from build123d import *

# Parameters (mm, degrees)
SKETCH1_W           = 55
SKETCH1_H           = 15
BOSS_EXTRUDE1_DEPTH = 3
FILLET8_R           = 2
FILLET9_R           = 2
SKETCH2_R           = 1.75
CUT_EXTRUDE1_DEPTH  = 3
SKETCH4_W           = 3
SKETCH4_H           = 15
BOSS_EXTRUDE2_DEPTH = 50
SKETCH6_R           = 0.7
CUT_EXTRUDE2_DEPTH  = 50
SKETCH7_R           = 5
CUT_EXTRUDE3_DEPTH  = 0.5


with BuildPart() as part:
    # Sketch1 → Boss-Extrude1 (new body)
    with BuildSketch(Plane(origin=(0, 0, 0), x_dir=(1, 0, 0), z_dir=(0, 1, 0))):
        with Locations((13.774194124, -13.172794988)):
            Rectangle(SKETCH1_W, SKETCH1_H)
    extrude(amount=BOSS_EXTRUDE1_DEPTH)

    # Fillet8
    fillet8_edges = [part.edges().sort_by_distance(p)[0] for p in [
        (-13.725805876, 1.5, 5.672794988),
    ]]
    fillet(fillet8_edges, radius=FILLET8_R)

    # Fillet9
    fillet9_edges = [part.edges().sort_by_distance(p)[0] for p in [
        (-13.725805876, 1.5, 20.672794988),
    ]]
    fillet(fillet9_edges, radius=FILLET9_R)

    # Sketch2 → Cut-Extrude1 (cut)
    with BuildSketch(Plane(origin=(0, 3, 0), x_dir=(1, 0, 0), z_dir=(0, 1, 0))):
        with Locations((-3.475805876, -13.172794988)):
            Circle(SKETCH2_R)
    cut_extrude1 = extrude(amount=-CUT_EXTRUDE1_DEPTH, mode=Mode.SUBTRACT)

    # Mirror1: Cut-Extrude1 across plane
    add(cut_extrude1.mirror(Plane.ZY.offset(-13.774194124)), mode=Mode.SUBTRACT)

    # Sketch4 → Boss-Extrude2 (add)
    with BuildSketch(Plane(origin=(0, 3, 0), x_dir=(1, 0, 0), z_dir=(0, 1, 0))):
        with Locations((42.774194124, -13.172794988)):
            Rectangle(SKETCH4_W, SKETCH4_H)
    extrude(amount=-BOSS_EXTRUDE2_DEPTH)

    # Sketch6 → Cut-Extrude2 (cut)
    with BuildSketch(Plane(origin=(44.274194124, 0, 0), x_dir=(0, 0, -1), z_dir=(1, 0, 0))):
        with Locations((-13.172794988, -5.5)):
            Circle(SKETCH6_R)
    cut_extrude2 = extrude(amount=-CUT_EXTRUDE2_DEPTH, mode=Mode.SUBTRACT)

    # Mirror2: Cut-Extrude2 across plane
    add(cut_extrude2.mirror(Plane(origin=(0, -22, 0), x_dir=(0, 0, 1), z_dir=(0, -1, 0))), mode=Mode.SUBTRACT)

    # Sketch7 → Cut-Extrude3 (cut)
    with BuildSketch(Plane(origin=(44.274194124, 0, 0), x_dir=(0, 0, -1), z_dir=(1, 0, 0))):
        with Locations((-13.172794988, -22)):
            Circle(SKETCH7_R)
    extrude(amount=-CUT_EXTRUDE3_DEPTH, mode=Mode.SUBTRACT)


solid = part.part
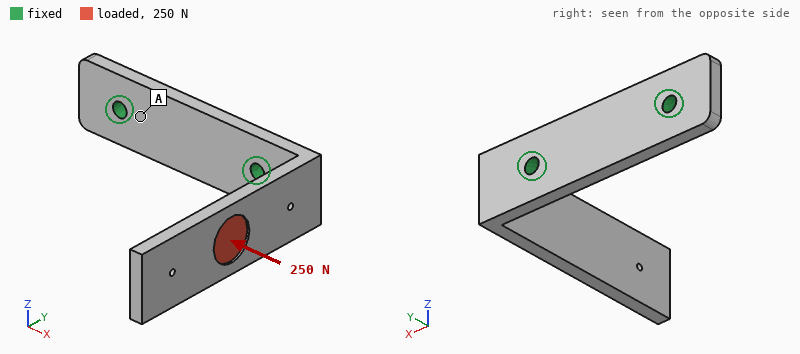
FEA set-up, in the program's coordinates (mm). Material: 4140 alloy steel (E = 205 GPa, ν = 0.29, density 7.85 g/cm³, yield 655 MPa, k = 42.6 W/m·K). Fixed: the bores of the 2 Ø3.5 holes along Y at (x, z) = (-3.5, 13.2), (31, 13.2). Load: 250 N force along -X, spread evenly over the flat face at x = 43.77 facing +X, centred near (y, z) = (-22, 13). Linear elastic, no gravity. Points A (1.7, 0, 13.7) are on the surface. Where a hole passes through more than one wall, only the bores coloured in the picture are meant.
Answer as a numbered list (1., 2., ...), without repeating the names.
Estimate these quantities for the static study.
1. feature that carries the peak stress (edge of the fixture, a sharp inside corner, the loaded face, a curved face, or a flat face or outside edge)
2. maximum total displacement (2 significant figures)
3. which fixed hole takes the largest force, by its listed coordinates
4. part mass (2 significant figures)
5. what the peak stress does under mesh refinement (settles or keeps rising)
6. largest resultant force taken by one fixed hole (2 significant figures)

1. edge of the fixture
2. 0.83 mm
3. (31, 13.2)
4. 36 g
5. keeps rising
6. 230 N
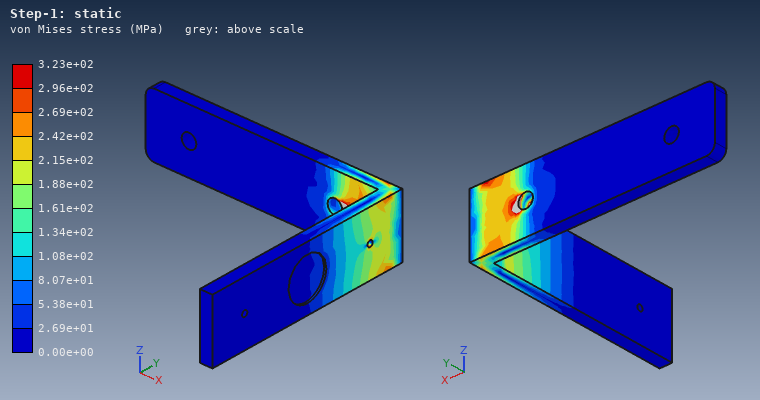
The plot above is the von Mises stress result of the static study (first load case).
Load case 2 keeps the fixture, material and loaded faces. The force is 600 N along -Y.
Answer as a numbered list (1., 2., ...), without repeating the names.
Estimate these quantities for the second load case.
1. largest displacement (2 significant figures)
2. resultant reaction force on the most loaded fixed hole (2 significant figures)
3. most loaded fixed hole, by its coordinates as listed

1. 0.40 mm
2. 620 N
3. (31, 13.2)
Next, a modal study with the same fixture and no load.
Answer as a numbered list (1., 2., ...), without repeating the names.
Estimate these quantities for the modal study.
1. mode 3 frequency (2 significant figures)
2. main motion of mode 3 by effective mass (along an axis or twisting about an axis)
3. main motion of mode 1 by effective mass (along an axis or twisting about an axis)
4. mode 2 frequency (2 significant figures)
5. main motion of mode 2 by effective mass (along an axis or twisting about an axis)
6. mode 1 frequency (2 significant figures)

1. 4400 Hz
2. along Y
3. along X
4. 1400 Hz
5. along Z
6. 770 Hz
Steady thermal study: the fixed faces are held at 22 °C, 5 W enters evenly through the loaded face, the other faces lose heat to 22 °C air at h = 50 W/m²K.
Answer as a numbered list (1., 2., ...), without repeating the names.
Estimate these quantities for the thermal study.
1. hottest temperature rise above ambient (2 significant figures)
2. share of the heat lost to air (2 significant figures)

1. 46 K
2. 59 %
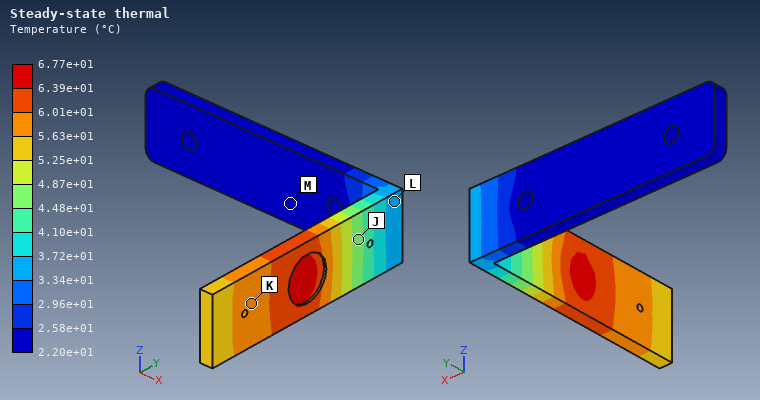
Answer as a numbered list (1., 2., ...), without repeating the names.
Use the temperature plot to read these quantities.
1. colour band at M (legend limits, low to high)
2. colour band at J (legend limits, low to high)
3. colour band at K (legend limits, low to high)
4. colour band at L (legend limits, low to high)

1. 2.20e+01 to 2.58e+01 °C
2. 4.48e+01 to 4.87e+01 °C
3. 5.63e+01 to 6.01e+01 °C
4. 3.34e+01 to 3.72e+01 °C
